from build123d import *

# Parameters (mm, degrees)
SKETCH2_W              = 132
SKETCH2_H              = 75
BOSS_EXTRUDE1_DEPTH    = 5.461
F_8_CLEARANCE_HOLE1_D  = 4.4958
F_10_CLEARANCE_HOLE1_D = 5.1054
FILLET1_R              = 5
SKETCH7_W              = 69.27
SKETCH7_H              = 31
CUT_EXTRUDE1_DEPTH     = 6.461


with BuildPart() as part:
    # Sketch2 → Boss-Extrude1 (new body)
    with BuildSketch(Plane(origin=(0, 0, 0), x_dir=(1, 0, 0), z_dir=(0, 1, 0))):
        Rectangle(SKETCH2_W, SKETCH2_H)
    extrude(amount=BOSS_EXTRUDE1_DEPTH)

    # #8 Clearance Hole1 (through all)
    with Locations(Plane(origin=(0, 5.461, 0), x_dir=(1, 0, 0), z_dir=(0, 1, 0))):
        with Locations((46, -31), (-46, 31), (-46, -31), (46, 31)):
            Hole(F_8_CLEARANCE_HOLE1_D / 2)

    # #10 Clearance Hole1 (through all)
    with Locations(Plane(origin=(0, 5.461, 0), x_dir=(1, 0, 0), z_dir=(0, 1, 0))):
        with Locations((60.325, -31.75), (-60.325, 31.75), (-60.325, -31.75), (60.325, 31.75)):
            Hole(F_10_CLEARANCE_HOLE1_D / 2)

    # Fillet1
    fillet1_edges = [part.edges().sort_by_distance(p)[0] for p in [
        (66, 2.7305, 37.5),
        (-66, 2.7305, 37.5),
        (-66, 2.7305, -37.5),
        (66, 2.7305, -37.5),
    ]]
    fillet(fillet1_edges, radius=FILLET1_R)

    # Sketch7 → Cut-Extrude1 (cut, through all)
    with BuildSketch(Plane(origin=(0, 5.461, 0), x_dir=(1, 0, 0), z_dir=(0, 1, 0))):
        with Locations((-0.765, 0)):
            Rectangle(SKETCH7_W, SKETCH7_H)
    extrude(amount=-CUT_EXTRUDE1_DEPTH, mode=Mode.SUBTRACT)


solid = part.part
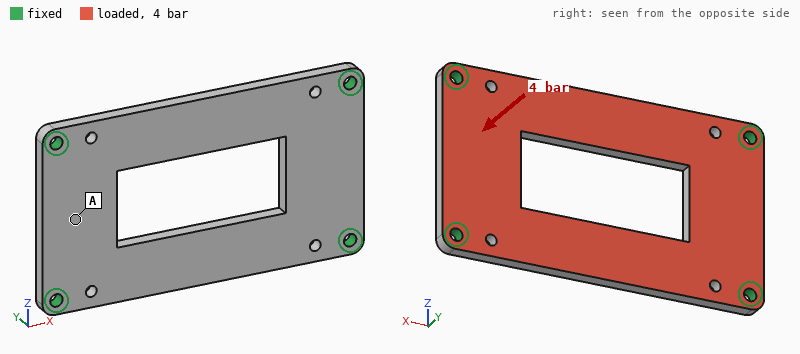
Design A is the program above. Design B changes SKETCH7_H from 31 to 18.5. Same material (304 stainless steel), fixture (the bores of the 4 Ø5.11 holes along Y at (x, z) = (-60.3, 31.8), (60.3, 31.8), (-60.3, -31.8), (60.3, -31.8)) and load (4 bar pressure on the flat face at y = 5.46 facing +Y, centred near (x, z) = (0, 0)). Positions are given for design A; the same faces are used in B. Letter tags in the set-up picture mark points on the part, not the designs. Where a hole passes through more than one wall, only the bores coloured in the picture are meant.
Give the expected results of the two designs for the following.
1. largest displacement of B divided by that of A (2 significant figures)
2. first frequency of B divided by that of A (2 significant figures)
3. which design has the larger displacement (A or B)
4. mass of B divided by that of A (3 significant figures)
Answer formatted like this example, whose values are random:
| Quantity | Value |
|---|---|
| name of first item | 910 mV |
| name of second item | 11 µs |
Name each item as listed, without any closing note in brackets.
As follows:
| Quantity | Value |
|---|---|
| largest displacement of B divided by that of A | 1.2 |
| first frequency of B divided by that of A | 0.93 |
| which design has the larger displacement | B |
| mass of B divided by that of A | 1.11 |
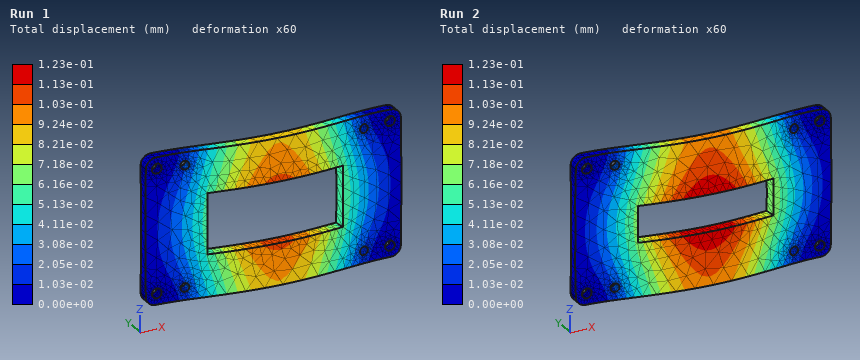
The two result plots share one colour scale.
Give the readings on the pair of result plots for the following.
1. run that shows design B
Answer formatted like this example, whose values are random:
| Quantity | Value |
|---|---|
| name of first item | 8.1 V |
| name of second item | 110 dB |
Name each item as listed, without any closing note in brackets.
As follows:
| Quantity | Value |
|---|---|
| run that shows design B | Run 2 |
